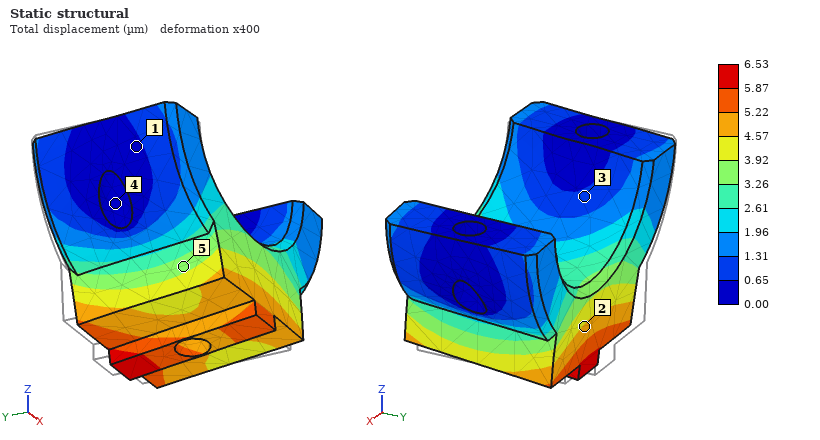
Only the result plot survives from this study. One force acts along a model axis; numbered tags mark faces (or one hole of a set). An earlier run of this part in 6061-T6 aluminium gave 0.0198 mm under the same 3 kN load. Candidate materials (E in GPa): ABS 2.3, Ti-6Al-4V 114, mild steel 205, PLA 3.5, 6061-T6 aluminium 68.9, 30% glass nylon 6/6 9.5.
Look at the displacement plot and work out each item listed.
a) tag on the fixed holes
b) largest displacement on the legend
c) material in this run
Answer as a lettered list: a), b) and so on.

a) 4
b) 6.53 µm
c) mild steel
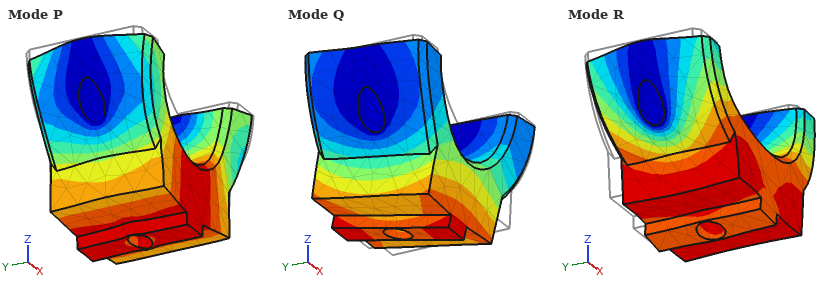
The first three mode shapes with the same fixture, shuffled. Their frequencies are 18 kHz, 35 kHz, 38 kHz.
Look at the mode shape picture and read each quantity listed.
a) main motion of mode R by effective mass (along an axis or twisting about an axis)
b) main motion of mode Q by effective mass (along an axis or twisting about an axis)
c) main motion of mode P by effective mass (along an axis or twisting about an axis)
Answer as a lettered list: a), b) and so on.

a) along X
b) along Y
c) along Z
